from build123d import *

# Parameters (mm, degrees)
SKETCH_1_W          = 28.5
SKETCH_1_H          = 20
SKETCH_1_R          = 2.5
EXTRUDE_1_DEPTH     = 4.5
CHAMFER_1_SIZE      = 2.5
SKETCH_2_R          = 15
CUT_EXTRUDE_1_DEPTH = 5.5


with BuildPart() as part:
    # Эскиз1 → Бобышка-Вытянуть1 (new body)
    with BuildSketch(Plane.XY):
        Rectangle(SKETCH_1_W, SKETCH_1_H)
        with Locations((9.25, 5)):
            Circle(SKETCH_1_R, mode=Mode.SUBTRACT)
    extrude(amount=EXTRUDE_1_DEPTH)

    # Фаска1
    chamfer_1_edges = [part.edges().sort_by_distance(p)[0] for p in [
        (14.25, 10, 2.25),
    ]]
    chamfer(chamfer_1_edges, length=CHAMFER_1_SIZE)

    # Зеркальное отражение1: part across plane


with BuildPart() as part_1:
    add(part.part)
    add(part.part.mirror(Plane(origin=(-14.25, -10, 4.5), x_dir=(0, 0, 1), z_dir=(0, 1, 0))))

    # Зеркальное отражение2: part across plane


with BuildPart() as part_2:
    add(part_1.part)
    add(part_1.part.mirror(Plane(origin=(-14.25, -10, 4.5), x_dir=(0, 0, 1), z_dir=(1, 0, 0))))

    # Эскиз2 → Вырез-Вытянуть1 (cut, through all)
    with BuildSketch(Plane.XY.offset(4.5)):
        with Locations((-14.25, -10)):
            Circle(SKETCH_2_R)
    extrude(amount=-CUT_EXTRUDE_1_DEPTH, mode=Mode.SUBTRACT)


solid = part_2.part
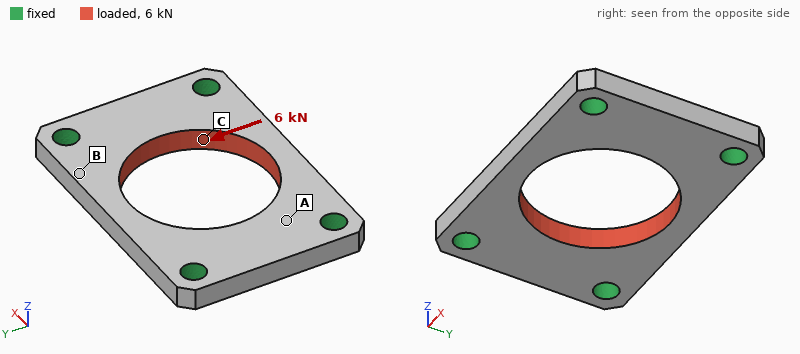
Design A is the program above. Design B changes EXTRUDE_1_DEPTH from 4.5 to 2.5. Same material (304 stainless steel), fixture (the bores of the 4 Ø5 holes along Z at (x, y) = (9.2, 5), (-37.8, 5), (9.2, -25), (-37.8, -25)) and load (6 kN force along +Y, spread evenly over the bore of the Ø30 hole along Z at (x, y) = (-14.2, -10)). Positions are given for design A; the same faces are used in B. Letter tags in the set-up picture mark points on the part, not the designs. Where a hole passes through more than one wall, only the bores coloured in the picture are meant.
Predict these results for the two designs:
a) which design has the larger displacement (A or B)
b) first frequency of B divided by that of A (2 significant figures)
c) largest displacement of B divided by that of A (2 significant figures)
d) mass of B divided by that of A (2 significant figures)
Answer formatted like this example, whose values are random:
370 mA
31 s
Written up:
B
0.60
1.8
0.56
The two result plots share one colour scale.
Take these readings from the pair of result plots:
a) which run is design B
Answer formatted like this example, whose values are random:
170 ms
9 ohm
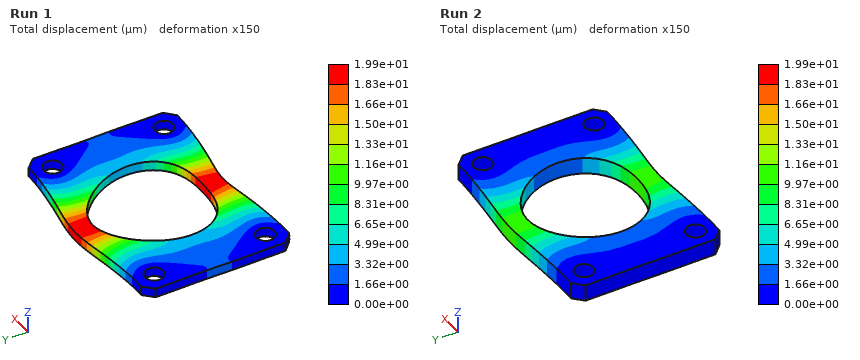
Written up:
Run 1
